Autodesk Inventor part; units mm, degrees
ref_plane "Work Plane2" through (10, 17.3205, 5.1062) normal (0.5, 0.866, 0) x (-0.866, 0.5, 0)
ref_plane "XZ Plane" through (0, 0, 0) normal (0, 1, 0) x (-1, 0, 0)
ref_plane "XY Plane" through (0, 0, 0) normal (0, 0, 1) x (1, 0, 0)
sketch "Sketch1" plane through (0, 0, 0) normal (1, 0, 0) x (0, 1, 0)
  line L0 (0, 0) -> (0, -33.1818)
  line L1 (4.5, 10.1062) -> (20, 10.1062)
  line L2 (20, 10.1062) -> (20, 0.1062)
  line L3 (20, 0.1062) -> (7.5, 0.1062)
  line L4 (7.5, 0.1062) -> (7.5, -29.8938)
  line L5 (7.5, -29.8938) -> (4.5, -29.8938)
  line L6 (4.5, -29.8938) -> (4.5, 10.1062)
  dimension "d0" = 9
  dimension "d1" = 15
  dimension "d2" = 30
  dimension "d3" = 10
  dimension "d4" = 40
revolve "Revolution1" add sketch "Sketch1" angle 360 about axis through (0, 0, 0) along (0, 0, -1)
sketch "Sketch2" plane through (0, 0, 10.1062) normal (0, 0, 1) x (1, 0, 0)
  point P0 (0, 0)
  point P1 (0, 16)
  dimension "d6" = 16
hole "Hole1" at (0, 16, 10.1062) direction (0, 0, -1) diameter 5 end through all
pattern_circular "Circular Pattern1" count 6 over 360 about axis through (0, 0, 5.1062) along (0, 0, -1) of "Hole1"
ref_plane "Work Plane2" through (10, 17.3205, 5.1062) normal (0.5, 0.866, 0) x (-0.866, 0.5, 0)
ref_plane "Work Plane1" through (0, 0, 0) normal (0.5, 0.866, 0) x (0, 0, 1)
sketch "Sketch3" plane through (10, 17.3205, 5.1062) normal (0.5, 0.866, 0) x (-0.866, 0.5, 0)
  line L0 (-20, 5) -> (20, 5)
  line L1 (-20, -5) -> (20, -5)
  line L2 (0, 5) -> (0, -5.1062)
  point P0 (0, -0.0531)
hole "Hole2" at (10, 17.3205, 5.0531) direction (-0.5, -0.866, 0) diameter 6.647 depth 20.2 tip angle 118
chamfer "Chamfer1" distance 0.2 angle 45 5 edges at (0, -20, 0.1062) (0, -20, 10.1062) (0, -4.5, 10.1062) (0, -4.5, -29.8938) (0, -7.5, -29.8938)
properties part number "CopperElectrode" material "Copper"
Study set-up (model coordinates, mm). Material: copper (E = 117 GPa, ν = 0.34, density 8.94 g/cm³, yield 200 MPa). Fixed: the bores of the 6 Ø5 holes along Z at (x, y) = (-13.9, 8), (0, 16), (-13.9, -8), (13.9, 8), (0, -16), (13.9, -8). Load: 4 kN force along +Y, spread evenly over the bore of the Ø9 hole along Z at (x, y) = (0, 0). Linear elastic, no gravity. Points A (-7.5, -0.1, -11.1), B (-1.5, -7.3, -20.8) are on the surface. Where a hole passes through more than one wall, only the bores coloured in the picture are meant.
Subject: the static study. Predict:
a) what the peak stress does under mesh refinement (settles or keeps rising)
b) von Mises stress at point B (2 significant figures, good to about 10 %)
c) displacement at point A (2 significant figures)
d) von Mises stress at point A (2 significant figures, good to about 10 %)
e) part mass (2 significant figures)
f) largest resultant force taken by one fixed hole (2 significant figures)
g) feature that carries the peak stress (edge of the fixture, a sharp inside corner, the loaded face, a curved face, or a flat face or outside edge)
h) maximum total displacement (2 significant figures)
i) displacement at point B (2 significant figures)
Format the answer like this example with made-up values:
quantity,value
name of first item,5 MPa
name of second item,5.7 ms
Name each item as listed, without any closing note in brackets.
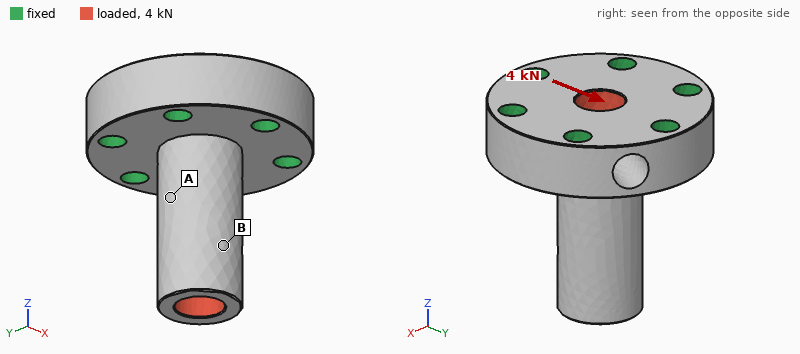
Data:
quantity,value
what the peak stress does under mesh refinement,keeps rising
von Mises stress at point B,15 MPa
displacement at point A,29 µm
von Mises stress at point A,49 MPa
part mass,120 g
largest resultant force taken by one fixed hole,2.0 kN
feature that carries the peak stress,a sharp inside corner
maximum total displacement,87 µm
displacement at point B,62 µm
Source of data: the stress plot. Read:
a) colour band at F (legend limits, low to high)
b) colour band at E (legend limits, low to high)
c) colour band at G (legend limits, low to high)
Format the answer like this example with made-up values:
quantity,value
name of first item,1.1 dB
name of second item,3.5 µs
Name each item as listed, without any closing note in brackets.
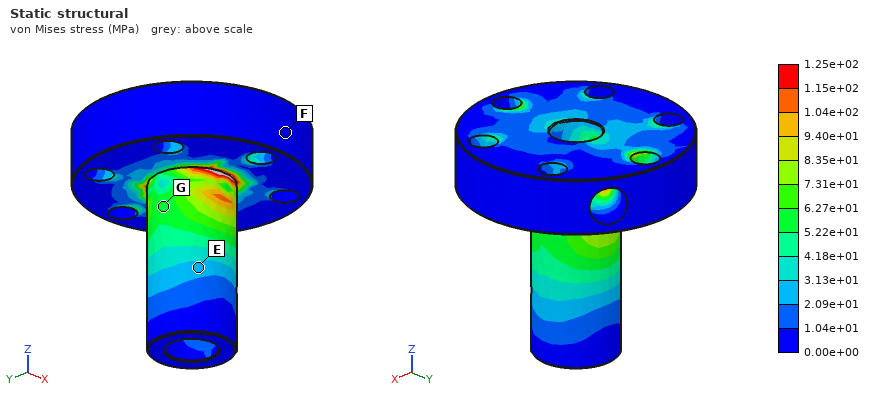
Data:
quantity,value
colour band at F,0.00e+00 to 1.04e+01 MPa
colour band at E,2.09e+01 to 3.13e+01 MPa
colour band at G,5.22e+01 to 6.27e+01 MPa
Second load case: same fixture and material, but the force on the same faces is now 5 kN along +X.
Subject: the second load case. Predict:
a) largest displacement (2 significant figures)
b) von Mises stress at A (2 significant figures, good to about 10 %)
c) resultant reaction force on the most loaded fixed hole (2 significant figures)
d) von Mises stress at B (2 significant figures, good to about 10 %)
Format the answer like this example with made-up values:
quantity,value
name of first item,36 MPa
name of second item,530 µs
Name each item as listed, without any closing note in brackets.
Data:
quantity,value
largest displacement,0.11 mm
von Mises stress at A,76 MPa
resultant reaction force on the most loaded fixed hole,2.3 kN
von Mises stress at B,29 MPa
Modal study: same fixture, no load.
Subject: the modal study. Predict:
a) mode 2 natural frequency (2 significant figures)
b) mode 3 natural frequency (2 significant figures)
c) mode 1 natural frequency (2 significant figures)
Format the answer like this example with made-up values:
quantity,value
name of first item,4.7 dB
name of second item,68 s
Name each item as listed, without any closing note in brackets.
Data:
quantity,value
mode 2 natural frequency,6600 Hz
mode 3 natural frequency,17 kHz
mode 1 natural frequency,6500 Hz
